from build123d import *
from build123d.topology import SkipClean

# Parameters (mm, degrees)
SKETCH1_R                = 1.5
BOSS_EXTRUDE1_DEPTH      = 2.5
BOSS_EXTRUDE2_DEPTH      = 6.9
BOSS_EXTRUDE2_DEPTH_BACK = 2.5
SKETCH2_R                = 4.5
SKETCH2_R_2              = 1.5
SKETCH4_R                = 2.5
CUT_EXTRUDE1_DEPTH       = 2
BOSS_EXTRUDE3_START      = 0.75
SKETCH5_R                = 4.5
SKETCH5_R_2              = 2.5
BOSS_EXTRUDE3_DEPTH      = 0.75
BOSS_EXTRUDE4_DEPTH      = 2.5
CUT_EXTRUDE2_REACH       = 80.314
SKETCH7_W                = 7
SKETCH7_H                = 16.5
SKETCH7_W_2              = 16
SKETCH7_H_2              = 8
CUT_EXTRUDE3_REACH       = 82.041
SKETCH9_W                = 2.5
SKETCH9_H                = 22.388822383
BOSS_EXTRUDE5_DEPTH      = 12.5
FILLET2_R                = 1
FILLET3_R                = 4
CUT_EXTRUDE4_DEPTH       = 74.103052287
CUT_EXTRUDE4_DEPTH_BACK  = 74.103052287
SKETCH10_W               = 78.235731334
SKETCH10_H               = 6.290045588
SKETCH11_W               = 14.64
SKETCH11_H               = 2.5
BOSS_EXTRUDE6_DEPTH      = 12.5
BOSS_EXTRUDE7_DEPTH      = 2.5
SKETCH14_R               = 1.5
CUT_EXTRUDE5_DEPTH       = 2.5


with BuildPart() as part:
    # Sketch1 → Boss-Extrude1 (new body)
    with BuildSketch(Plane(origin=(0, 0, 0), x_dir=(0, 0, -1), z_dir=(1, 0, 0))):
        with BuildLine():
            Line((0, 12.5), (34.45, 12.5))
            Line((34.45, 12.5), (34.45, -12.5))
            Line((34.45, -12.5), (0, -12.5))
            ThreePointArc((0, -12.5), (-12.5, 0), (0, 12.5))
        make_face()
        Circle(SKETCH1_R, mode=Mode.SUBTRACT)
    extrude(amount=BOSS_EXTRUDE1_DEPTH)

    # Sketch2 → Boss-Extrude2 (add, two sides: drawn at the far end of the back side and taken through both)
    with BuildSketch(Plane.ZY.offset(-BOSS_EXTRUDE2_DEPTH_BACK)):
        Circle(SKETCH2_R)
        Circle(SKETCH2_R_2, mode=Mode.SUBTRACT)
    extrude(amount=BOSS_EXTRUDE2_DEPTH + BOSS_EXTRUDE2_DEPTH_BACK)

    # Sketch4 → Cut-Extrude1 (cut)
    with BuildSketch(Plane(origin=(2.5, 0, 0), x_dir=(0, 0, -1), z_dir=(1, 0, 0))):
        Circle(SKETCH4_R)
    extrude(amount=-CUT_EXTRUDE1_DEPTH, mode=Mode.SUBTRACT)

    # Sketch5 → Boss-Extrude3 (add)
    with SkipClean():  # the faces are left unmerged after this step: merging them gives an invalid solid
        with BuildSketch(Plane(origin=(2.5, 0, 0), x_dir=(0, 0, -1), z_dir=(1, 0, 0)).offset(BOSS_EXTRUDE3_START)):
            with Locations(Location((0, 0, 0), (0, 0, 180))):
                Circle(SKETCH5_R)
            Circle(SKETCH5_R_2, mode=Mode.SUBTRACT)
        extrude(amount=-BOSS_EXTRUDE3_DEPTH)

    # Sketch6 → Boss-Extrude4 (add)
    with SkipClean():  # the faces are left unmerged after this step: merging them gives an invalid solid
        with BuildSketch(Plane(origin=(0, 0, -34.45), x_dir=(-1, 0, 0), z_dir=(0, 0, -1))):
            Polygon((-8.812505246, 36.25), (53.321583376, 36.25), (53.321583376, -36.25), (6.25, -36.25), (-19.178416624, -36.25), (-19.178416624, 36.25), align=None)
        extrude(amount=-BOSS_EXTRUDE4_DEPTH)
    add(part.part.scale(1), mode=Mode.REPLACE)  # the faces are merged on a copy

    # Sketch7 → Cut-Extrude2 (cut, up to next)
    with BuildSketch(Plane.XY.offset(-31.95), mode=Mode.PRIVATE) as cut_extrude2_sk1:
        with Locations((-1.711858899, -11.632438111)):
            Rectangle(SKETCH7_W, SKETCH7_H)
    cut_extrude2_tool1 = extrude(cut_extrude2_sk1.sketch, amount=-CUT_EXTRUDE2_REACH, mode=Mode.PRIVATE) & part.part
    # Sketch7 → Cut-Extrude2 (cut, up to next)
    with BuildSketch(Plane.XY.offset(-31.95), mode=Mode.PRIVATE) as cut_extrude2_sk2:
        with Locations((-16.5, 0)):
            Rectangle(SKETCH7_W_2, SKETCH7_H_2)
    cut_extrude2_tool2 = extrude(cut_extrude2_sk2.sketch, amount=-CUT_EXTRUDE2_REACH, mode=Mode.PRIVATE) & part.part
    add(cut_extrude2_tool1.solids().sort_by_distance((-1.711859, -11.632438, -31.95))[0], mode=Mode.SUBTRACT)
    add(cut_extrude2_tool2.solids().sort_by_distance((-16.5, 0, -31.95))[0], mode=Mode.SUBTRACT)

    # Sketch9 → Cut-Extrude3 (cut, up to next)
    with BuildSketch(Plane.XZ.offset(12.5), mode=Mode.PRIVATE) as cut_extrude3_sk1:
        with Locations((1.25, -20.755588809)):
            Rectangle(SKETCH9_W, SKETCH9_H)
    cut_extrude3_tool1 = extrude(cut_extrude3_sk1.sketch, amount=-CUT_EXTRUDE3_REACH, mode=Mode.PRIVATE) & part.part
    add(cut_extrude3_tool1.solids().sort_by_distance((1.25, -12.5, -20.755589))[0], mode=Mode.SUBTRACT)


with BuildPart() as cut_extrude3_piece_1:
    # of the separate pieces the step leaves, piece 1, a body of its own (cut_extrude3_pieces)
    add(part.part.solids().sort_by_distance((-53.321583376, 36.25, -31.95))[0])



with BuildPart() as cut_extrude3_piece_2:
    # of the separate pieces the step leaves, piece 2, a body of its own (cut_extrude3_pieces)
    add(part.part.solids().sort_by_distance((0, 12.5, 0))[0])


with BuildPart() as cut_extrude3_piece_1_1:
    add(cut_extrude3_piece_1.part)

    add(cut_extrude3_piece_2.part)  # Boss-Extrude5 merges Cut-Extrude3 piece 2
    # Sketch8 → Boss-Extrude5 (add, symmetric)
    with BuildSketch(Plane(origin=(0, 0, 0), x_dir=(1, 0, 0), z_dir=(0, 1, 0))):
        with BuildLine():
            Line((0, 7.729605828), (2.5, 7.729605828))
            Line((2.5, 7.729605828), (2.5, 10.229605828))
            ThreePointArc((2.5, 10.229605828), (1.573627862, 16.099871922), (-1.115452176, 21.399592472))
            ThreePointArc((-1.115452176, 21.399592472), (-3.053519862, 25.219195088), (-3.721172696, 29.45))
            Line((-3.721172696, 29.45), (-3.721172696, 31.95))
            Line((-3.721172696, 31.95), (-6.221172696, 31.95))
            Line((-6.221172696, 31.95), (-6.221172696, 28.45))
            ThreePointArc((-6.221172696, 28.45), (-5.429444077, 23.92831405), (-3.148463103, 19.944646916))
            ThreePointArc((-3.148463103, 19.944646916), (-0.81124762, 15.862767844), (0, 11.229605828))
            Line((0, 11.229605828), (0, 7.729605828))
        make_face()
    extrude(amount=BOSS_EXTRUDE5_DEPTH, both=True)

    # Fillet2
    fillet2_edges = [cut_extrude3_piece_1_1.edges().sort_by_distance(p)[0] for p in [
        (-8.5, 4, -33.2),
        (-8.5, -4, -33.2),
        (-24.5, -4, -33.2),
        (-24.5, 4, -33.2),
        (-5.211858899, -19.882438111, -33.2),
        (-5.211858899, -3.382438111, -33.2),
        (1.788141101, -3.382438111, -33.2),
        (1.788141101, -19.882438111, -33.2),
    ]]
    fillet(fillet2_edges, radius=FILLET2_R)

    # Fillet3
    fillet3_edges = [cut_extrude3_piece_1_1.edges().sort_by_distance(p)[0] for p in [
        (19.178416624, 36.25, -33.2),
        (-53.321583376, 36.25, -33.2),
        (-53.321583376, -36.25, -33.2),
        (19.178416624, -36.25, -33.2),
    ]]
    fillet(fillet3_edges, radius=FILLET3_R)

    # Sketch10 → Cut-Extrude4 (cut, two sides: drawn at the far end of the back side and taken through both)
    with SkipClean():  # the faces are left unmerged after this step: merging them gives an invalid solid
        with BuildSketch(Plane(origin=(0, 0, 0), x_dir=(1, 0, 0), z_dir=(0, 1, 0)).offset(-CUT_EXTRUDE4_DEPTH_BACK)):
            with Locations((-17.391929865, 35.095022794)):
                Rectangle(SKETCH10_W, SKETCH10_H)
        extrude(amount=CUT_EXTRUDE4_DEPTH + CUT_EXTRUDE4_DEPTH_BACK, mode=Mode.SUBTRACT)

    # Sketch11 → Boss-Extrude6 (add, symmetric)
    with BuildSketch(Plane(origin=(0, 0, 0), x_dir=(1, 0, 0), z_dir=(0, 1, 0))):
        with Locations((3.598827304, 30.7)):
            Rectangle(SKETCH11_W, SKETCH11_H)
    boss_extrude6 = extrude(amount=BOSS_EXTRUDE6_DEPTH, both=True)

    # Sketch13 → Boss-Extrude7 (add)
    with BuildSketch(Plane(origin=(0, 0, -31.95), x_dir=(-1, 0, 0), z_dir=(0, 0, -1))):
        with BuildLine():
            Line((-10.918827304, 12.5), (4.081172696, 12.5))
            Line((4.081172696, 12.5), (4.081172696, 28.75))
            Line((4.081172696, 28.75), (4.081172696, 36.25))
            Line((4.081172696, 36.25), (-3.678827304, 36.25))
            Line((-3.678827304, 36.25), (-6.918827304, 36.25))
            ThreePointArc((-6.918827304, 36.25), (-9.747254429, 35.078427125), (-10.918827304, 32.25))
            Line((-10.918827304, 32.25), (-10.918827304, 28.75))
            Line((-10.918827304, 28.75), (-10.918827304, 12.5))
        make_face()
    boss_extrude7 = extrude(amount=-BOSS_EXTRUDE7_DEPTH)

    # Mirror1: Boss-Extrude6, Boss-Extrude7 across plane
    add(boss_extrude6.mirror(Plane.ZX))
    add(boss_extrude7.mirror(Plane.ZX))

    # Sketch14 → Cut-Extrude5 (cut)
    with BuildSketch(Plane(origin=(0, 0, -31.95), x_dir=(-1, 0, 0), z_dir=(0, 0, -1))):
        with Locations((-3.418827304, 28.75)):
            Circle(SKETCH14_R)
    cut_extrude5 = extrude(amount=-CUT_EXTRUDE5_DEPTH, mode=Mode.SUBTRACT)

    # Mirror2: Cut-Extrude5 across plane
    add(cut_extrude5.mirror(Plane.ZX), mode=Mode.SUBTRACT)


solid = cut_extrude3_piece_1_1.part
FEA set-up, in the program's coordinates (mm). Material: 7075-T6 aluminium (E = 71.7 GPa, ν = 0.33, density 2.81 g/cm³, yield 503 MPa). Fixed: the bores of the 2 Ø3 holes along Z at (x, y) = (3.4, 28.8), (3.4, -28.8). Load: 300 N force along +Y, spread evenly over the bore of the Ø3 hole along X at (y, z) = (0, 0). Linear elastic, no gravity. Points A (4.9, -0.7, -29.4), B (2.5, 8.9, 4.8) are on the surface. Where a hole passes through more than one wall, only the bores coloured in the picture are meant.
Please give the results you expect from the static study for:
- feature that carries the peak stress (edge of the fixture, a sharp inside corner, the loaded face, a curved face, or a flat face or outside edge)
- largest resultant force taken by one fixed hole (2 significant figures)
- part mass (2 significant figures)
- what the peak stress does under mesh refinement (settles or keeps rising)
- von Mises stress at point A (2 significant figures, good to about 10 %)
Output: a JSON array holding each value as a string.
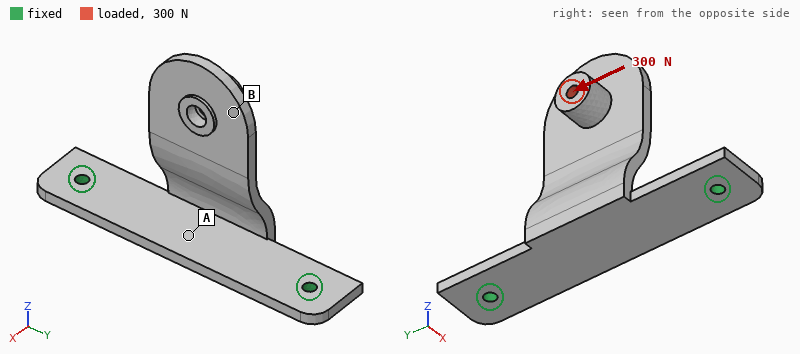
["a sharp inside corner", "270 N", "16 g", "keeps rising", "52 MPa"]
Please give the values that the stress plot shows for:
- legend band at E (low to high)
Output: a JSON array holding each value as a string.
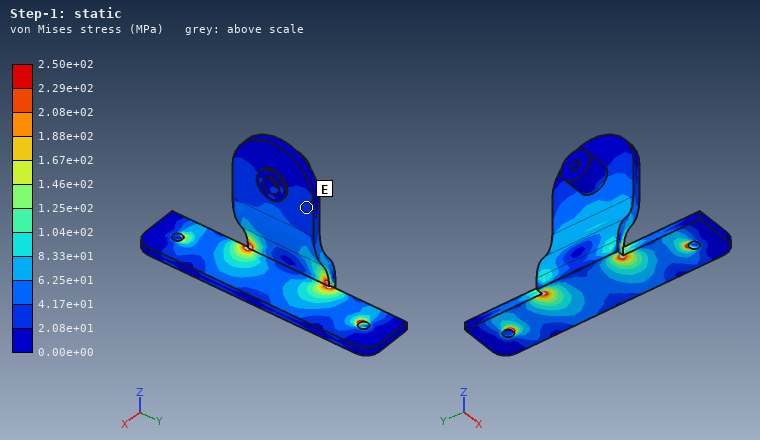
["2.08e+01 to 4.17e+01 MPa"]
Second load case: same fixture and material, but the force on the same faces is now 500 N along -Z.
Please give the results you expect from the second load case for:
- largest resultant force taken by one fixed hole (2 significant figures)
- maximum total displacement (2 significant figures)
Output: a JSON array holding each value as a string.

["260 N", "0.95 mm"]
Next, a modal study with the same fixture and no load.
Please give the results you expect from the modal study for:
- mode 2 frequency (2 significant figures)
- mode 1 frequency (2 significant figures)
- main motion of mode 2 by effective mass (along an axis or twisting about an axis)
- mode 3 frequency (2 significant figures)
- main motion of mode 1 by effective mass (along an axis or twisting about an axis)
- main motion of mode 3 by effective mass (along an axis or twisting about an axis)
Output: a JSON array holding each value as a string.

["1900 Hz", "700 Hz", "along Y", "2400 Hz", "along X", "along Z"]
